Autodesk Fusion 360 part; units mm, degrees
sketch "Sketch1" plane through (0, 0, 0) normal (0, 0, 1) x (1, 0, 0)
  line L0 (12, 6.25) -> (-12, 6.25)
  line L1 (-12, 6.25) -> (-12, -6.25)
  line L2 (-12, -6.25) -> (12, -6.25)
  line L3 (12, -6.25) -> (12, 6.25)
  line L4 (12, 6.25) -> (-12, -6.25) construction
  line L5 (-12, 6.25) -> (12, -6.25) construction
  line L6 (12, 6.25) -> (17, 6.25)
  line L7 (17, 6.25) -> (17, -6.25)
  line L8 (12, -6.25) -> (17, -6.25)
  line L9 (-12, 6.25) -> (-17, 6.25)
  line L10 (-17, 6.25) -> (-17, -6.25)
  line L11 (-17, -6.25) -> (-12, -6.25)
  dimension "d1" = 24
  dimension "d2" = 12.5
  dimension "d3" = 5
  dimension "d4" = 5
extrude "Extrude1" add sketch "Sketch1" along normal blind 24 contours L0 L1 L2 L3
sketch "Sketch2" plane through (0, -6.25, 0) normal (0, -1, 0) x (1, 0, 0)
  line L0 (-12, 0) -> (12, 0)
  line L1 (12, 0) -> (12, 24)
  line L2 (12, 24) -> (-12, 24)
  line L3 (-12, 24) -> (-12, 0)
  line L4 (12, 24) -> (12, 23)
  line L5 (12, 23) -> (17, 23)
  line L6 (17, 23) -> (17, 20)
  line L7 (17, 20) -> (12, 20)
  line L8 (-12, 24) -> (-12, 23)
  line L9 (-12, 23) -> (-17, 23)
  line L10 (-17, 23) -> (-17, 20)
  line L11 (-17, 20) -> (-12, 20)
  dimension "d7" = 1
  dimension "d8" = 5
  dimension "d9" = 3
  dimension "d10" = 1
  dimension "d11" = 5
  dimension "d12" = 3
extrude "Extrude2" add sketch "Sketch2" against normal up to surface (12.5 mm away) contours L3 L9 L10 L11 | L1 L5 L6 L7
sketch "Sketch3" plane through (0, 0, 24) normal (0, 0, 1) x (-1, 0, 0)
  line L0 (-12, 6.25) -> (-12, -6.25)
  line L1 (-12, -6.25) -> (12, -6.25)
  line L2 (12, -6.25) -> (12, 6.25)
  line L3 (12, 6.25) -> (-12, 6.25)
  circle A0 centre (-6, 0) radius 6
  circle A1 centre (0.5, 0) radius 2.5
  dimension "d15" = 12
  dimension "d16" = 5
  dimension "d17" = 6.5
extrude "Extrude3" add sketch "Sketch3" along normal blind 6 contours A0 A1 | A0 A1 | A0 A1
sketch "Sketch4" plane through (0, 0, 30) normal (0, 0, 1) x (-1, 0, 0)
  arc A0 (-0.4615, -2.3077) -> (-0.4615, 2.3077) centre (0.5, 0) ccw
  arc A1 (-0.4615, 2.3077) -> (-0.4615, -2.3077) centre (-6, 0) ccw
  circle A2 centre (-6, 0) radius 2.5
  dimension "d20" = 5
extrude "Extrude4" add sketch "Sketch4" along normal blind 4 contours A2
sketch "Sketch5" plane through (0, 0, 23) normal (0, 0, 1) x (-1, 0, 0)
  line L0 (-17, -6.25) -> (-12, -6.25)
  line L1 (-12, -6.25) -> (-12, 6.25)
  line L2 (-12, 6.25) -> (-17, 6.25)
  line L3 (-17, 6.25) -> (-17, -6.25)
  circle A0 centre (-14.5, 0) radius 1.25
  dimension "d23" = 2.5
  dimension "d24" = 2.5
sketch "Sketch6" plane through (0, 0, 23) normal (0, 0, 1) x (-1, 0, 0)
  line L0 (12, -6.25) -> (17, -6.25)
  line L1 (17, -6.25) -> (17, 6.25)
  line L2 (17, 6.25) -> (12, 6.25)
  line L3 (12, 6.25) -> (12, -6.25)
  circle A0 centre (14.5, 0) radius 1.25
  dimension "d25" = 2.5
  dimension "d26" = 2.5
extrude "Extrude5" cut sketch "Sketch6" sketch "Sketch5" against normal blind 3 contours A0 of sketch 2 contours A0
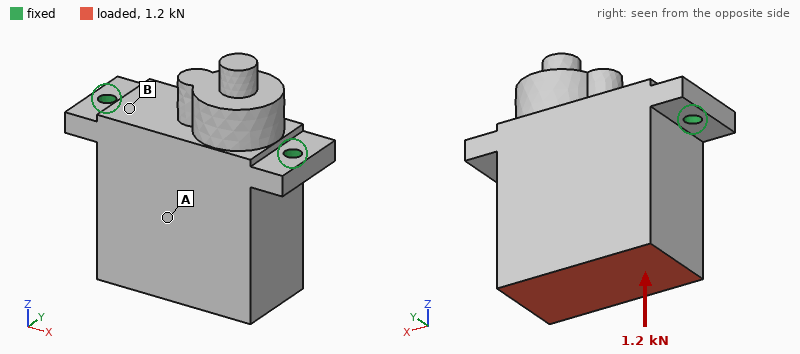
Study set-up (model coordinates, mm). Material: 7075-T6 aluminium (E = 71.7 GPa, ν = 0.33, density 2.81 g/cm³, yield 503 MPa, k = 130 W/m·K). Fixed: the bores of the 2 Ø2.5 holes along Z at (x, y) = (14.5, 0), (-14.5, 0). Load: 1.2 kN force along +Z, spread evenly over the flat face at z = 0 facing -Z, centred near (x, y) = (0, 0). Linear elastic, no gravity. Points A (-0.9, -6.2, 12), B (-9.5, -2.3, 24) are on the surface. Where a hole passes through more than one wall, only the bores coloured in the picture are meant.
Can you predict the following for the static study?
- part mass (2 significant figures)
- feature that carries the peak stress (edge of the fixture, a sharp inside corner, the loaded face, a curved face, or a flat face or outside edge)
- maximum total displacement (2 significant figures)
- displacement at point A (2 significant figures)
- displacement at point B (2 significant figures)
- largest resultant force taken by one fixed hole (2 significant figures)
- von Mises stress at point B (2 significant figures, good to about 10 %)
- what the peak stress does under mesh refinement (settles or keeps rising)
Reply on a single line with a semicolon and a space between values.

24 g; edge of the fixture; 6.6 µm; 5.9 µm; 4.9 µm; 620 N; 17 MPa; keeps rising
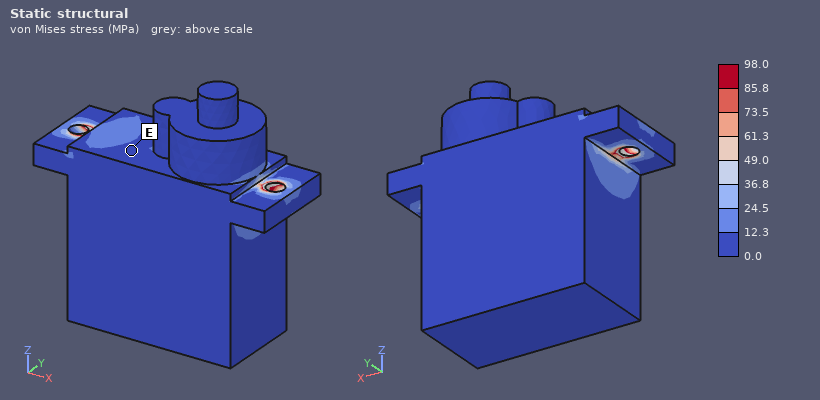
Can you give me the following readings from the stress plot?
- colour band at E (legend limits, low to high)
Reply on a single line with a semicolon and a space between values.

0.0 to 12.3 MPa
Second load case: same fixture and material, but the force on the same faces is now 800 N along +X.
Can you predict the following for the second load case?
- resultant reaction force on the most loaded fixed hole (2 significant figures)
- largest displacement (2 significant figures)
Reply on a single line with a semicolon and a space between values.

790 N; 15 µm
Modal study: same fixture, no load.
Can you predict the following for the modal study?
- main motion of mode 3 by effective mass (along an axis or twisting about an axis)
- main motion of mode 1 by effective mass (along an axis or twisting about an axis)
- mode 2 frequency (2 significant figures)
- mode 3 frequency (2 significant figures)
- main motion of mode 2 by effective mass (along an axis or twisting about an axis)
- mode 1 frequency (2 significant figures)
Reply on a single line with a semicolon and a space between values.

along Z; along Y; 14 kHz; 16 kHz; along X; 3700 Hz
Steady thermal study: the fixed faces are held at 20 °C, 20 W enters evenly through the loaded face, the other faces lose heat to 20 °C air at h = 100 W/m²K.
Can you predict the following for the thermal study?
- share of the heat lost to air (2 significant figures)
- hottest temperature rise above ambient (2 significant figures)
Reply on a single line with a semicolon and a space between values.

15 %; 19 K
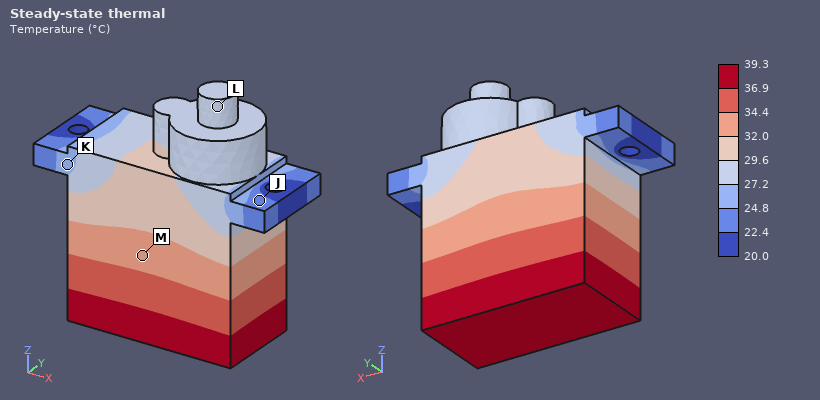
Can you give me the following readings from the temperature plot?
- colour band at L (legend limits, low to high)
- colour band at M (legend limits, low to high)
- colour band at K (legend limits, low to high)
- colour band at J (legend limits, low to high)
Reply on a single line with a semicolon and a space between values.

27.2 to 29.6 °C; 32.0 to 34.4 °C; 24.8 to 27.2 °C; 22.4 to 24.8 °C
